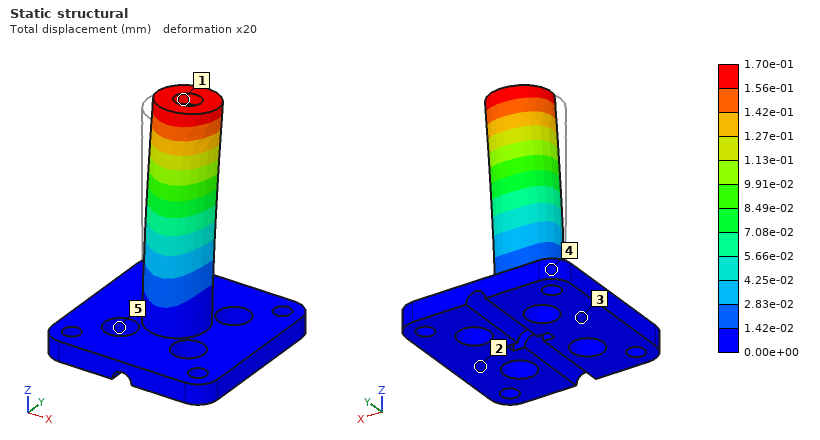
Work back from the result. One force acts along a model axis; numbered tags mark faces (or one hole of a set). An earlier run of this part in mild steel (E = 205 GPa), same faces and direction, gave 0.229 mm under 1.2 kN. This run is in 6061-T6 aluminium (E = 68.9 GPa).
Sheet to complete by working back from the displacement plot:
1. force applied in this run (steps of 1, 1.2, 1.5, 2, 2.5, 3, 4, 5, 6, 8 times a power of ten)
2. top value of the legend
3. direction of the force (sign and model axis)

300 N
1.70e-01 mm
+Y
